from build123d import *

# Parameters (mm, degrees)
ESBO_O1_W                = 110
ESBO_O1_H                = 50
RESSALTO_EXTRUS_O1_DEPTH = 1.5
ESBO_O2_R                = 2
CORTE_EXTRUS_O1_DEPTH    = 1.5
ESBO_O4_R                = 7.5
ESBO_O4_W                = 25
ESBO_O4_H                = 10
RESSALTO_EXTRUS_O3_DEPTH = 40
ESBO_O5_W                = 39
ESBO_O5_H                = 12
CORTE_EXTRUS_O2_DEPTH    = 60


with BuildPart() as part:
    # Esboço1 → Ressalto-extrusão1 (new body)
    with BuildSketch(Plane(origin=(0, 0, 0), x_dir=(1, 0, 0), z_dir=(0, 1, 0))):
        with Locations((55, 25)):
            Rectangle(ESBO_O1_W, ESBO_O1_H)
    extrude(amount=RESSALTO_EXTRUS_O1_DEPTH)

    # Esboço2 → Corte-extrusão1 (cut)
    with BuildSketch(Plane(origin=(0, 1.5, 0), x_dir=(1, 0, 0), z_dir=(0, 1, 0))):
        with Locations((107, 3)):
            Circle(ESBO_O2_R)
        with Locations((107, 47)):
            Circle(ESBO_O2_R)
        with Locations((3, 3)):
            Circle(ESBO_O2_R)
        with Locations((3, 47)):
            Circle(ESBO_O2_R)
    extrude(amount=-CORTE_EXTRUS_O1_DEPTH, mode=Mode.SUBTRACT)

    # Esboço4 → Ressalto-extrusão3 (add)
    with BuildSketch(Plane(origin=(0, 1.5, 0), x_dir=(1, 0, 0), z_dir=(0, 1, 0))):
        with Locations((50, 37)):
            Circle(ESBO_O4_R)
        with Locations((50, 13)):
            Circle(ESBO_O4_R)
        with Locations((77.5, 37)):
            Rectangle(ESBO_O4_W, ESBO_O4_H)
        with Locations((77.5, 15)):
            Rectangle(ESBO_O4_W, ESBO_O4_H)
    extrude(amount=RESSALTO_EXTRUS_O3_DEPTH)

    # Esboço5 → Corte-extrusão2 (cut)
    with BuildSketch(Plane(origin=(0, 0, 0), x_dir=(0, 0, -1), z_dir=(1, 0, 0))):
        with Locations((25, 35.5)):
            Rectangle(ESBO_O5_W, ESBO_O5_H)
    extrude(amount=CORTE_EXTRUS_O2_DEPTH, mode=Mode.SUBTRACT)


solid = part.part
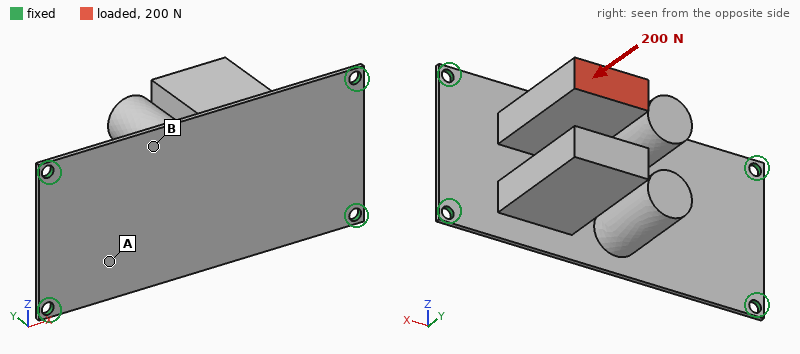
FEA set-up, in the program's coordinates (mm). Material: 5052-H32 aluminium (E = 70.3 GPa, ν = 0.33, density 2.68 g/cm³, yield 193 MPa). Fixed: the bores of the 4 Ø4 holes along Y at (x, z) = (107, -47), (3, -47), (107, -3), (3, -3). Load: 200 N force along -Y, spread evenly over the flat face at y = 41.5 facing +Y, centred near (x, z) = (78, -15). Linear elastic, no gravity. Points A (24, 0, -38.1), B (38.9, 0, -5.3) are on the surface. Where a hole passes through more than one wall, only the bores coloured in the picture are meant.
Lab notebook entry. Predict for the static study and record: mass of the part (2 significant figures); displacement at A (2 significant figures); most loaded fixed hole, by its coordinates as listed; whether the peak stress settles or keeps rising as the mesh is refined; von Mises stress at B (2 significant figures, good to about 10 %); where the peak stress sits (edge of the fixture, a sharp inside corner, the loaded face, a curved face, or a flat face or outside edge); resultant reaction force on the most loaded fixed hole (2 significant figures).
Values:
100 g
0.22 mm
(107, -3)
keeps rising
39 MPa
edge of the fixture
130 N
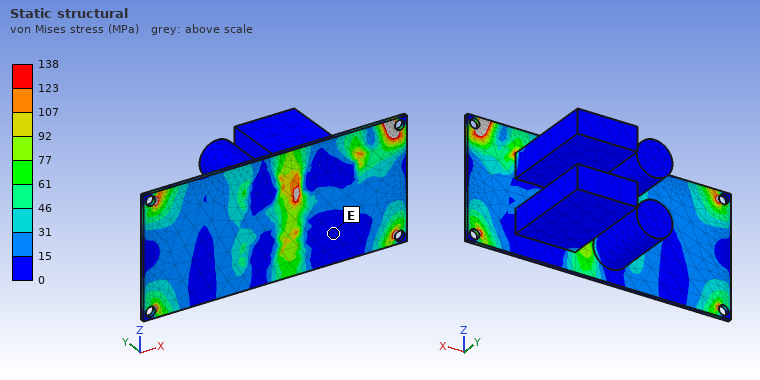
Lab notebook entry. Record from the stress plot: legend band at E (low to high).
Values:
0 to 15 MPa
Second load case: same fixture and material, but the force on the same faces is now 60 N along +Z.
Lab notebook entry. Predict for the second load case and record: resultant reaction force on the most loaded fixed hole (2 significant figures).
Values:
66 N
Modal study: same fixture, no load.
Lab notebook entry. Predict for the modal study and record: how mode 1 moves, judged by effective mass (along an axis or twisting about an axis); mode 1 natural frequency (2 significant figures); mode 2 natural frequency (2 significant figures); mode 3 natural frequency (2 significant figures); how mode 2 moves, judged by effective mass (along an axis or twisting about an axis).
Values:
along Y
270 Hz
430 Hz
570 Hz
along Z
